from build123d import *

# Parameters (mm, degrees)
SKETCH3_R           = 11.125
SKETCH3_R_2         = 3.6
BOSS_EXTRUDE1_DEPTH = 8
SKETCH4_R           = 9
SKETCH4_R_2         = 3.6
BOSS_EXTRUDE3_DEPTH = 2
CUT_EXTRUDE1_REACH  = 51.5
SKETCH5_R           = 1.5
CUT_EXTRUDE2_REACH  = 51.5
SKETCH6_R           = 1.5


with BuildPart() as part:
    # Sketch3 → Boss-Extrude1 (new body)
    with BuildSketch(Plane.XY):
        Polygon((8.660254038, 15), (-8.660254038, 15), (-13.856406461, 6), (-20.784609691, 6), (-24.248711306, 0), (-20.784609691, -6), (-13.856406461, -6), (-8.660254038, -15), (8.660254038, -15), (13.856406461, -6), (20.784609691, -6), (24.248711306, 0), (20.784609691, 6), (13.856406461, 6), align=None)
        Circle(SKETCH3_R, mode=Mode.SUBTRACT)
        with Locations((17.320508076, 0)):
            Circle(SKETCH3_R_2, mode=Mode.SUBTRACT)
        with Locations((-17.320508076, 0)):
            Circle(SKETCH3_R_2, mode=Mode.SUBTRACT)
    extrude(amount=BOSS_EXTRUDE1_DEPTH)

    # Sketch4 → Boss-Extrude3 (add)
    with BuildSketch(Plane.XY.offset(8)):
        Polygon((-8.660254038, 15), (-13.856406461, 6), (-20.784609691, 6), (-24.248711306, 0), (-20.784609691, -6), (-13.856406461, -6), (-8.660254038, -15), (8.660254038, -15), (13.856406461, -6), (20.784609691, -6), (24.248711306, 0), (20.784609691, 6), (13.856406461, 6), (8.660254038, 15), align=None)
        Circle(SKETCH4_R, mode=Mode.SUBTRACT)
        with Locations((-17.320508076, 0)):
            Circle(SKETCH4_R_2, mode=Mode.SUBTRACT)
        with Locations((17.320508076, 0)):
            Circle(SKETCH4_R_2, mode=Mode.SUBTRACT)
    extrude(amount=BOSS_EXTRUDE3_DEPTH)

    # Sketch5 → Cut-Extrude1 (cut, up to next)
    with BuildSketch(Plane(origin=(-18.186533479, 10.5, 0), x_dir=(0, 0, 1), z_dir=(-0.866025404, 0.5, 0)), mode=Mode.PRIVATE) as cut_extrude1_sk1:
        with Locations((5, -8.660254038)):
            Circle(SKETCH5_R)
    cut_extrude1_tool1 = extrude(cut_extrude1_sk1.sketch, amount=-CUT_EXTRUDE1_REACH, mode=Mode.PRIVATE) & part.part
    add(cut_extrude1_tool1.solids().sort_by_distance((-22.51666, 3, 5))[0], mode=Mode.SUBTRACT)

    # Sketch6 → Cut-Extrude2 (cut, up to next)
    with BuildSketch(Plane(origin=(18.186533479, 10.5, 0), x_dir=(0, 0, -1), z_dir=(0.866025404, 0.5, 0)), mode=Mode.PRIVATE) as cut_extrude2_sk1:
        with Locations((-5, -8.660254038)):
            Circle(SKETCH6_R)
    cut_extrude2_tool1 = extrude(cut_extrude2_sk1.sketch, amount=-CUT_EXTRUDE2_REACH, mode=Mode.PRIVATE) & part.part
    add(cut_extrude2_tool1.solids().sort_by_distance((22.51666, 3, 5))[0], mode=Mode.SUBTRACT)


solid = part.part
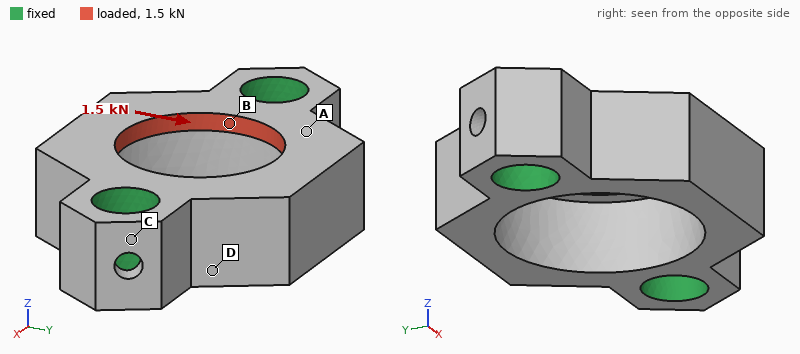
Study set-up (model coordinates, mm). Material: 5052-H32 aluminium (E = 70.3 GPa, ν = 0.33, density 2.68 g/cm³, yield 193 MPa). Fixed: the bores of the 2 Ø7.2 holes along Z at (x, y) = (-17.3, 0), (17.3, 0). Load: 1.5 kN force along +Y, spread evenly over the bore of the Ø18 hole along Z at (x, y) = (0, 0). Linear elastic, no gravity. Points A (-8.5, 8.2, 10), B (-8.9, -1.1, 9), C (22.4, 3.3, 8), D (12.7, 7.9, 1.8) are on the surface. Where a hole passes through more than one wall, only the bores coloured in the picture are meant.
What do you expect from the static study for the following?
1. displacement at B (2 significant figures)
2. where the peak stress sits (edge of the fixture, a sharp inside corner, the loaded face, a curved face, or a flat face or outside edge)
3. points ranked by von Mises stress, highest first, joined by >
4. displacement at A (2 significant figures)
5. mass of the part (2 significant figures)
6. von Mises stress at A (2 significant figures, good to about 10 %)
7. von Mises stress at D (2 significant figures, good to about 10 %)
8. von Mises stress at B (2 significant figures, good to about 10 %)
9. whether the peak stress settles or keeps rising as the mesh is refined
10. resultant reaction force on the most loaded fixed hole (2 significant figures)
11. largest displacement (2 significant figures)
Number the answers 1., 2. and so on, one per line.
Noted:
1. 3.4 µm
2. edge of the fixture
3. B > A > D > C
4. 4.6 µm
5. 13 g
6. 19 MPa
7. 7.5 MPa
8. 25 MPa
9. keeps rising
10. 750 N
11. 8.5 µm
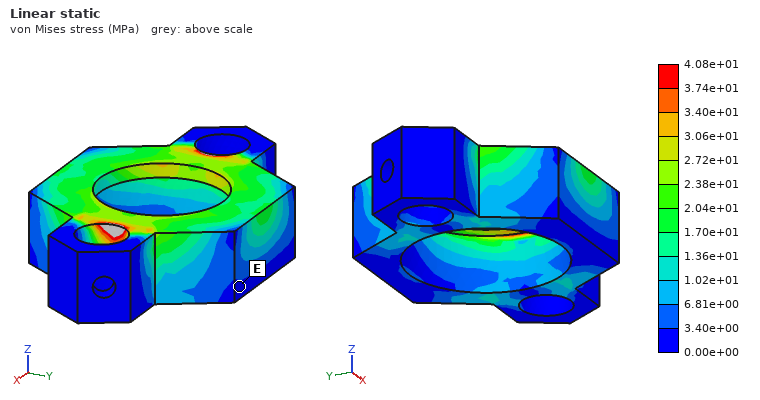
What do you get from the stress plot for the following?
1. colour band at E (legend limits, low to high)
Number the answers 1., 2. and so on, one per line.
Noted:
1. 0.00e+00 to 3.40e+00 MPa
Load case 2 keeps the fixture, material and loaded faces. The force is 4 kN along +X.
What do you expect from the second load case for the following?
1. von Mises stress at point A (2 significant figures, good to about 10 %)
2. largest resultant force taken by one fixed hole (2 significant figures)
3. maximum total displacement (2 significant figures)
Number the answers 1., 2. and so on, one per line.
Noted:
1. 35 MPa
2. 2.0 kN
3. 13 µm
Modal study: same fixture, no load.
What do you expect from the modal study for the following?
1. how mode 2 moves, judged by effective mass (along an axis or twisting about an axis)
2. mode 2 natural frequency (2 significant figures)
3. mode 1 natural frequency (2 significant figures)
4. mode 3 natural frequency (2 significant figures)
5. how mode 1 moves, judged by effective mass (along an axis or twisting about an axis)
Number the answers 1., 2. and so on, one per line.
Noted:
1. along Z
2. 22 kHz
3. 21 kHz
4. 33 kHz
5. twisting about X
